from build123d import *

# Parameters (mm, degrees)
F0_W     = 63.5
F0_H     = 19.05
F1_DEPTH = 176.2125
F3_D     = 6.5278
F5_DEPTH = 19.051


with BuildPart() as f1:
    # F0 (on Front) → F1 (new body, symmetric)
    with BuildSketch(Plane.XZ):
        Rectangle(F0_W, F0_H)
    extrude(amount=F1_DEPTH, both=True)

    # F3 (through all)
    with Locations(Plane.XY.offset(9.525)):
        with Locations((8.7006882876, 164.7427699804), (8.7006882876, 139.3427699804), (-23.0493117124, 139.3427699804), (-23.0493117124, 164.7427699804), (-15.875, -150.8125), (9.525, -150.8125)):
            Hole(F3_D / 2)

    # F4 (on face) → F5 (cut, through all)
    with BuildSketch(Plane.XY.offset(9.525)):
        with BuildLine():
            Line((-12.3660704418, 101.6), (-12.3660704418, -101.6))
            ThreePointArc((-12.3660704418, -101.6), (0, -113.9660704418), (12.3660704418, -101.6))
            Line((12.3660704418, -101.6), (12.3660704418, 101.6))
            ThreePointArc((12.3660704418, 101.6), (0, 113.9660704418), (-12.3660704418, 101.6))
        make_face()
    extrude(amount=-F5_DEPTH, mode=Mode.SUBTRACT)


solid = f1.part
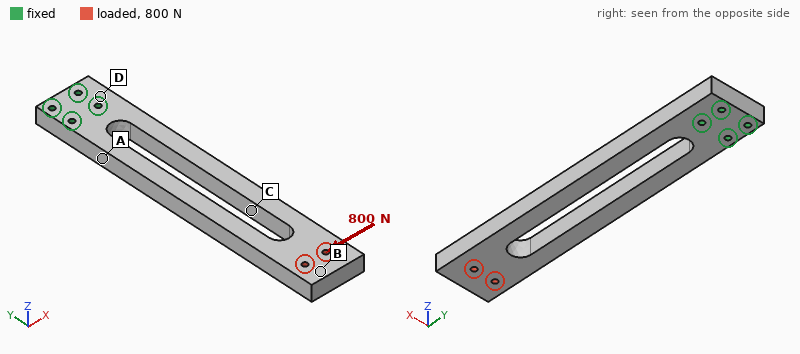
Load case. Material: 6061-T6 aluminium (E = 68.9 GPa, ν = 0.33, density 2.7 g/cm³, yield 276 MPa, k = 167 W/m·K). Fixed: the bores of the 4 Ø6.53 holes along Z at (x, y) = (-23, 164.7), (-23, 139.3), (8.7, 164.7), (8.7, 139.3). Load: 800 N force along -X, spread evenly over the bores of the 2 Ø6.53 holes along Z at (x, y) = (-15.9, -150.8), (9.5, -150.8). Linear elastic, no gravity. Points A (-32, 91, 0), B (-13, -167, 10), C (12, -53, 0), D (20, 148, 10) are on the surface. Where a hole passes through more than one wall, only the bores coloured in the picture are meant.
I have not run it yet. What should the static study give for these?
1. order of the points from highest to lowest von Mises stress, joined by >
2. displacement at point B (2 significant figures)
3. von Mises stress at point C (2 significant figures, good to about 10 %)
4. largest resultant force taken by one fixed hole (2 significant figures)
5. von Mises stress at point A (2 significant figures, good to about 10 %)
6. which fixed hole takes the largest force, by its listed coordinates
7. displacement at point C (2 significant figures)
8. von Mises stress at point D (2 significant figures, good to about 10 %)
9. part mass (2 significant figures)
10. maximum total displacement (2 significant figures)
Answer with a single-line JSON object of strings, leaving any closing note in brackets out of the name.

{"order of the points from highest to lowest von Mises stress, joined by >": "A > C > D > B", "displacement at point B": "0.80 mm", "von Mises stress at point C": "22 MPa", "largest resultant force taken by one fixed hole": "5.0 kN", "von Mises stress at point A": "40 MPa", "which fixed hole takes the largest force, by its listed coordinates": "(-23, 139.3)", "displacement at point C": "0.56 mm", "von Mises stress at point D": "10 MPa", "part mass": "860 g", "maximum total displacement": "0.82 mm"}
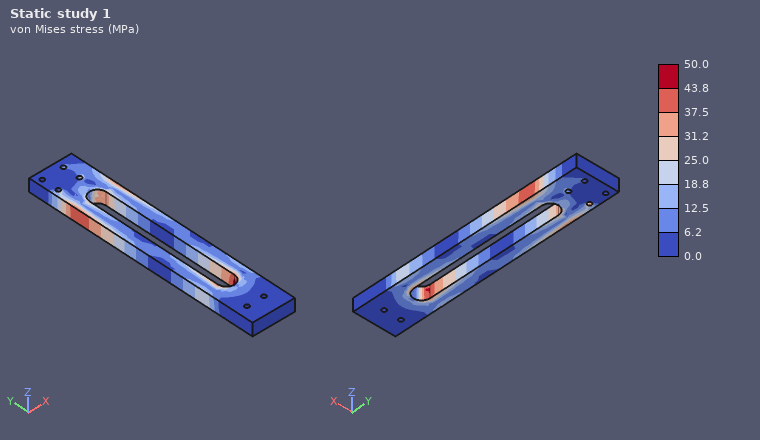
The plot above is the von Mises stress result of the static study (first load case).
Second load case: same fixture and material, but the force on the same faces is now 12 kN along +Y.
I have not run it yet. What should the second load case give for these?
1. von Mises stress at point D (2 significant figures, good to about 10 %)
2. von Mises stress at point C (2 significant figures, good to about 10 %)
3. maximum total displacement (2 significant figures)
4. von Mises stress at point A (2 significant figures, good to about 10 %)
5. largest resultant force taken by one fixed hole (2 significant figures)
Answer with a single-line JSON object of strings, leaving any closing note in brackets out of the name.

{"von Mises stress at point D": "8.2 MPa", "von Mises stress at point C": "17 MPa", "maximum total displacement": "92 µm", "von Mises stress at point A": "18 MPa", "largest resultant force taken by one fixed hole": "5.0 kN"}
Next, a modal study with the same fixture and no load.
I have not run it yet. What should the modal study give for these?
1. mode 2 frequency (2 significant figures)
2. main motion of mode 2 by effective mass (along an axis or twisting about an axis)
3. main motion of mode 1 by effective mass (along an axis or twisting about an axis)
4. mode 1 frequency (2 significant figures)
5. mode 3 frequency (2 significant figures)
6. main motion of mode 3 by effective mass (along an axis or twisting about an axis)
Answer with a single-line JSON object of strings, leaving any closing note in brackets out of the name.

{"mode 2 frequency": "280 Hz", "main motion of mode 2 by effective mass": "along X", "main motion of mode 1 by effective mass": "along Z", "mode 1 frequency": "140 Hz", "mode 3 frequency": "810 Hz", "main motion of mode 3 by effective mass": "twisting about Y"}
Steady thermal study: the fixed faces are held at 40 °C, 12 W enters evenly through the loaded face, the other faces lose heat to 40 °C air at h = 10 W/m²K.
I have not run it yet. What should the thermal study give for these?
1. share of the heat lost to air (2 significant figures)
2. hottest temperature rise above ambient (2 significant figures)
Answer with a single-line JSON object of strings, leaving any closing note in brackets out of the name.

{"share of the heat lost to air": "41 %", "hottest temperature rise above ambient": "18 K"}
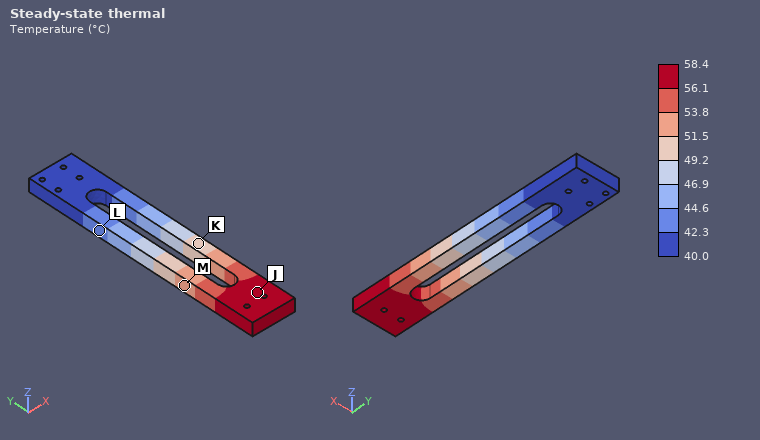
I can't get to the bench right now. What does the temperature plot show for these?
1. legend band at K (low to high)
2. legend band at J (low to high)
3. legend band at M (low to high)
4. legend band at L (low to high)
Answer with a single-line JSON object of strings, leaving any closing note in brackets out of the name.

{"legend band at K": "49.2 to 51.5 °C", "legend band at J": "56.1 to 58.4 °C", "legend band at M": "51.5 to 53.8 °C", "legend band at L": "42.3 to 44.6 °C"}
